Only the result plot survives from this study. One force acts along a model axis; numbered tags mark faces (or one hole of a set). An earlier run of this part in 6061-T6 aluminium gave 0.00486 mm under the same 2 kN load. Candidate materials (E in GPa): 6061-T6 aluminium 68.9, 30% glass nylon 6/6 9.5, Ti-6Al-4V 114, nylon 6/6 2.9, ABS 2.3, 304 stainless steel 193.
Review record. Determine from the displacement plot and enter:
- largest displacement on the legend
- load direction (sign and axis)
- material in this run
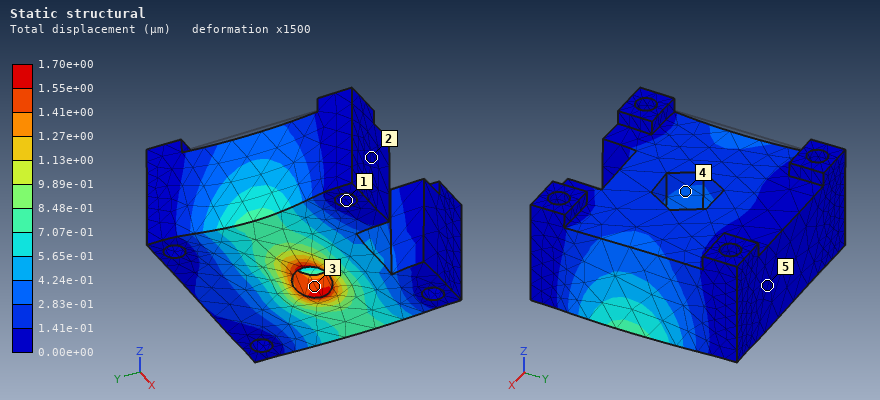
1.70e+00 µm
+X
304 stainless steel
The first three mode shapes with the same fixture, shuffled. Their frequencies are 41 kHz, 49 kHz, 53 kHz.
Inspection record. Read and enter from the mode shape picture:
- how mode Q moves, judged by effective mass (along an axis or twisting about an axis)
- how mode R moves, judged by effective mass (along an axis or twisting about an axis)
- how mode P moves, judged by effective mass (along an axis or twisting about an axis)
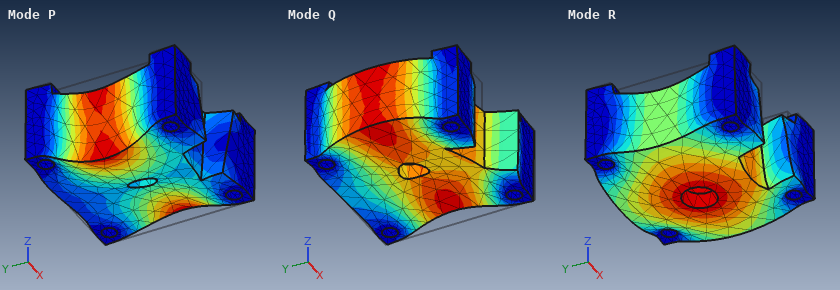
along X
along Z
twisting about Y
